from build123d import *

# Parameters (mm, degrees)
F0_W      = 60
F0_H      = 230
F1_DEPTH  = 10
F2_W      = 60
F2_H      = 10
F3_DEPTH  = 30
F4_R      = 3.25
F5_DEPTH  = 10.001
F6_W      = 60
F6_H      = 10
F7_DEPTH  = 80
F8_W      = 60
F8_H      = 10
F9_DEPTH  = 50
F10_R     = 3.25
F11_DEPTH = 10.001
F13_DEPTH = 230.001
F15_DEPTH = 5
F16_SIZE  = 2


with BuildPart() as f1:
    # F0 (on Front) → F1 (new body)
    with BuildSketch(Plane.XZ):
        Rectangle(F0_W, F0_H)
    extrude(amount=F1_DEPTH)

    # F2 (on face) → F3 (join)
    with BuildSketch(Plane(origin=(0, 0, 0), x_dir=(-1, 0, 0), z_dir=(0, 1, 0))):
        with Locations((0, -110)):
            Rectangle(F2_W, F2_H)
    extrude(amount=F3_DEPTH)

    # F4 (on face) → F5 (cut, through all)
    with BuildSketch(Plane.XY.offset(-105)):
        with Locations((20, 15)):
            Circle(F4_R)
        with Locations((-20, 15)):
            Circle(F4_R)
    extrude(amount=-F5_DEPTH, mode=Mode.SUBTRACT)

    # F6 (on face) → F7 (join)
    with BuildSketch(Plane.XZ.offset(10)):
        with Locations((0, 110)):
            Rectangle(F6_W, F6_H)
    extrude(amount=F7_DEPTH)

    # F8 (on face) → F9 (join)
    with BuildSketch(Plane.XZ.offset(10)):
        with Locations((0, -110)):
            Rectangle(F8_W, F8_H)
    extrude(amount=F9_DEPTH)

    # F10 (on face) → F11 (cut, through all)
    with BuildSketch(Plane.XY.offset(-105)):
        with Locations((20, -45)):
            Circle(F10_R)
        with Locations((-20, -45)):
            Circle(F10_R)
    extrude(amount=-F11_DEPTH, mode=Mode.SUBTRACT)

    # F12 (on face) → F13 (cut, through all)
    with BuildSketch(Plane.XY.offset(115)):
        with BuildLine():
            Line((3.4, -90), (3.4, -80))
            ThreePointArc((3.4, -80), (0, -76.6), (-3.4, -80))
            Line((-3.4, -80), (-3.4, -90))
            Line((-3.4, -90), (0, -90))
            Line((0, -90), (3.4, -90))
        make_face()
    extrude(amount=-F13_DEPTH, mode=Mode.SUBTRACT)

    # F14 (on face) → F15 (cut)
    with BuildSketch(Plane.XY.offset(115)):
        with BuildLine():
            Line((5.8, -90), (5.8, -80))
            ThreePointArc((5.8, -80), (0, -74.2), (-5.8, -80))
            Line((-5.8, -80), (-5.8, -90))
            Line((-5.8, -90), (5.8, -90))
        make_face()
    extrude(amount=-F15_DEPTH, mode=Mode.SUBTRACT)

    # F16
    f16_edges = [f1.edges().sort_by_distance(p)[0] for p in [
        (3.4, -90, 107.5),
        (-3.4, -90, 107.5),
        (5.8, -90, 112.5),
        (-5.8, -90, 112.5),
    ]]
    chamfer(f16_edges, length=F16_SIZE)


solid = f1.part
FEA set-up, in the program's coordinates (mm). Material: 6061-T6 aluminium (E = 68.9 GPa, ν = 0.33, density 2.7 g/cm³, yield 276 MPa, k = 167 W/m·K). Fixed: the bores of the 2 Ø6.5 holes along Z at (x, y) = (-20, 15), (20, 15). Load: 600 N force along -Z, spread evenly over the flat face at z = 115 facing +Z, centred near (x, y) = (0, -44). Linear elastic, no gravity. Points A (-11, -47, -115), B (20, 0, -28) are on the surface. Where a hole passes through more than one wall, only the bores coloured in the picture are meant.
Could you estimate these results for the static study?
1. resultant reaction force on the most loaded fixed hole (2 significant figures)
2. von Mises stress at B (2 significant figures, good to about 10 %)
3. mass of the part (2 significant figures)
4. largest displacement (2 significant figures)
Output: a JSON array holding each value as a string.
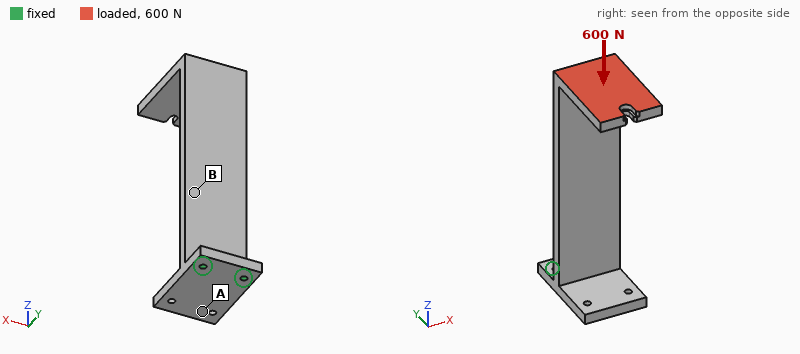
["310 N", "22 MPa", "620 g", "2.5 mm"]
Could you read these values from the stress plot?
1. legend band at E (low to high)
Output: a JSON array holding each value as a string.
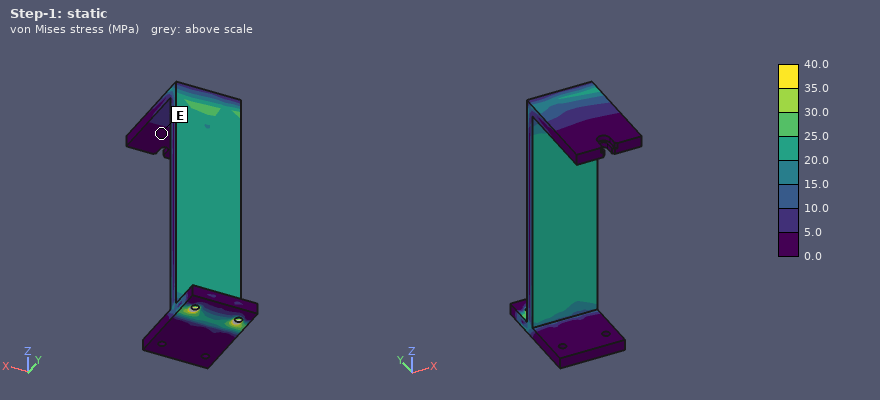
["0.0 to 5.0 MPa"]
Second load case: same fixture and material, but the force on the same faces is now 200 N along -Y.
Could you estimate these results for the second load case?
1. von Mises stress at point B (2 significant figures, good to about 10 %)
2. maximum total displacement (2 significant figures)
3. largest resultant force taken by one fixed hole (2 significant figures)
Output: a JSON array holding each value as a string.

["28 MPa", "3.0 mm", "160 N"]
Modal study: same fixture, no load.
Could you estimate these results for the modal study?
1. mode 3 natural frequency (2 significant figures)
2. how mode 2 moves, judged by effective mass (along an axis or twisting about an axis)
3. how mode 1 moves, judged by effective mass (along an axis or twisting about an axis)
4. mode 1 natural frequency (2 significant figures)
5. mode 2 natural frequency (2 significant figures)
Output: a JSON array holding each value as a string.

["510 Hz", "along X", "along Y", "93 Hz", "310 Hz"]
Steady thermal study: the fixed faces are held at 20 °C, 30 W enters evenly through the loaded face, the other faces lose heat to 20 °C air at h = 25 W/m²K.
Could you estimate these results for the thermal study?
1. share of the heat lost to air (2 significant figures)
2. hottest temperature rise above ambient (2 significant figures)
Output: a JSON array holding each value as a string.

["66 %", "41 K"]
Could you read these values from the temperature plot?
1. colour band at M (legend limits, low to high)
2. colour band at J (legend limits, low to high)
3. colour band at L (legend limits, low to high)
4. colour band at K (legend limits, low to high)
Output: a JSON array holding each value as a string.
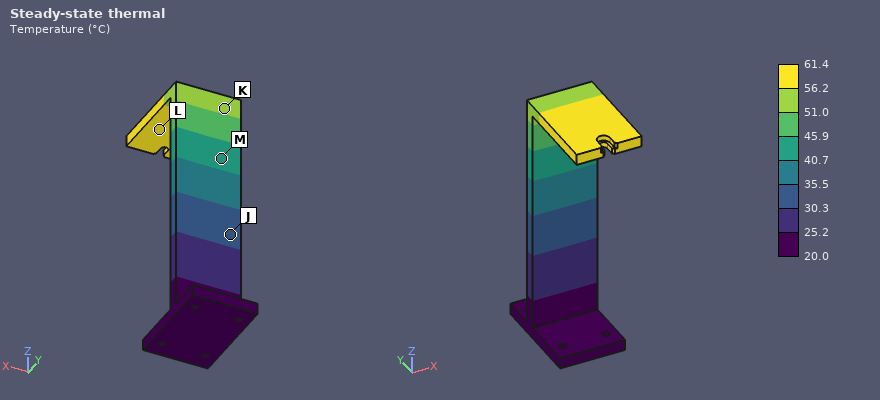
["40.7 to 45.9 °C", "30.3 to 35.5 °C", "56.2 to 61.4 °C", "51.0 to 56.2 °C"]
